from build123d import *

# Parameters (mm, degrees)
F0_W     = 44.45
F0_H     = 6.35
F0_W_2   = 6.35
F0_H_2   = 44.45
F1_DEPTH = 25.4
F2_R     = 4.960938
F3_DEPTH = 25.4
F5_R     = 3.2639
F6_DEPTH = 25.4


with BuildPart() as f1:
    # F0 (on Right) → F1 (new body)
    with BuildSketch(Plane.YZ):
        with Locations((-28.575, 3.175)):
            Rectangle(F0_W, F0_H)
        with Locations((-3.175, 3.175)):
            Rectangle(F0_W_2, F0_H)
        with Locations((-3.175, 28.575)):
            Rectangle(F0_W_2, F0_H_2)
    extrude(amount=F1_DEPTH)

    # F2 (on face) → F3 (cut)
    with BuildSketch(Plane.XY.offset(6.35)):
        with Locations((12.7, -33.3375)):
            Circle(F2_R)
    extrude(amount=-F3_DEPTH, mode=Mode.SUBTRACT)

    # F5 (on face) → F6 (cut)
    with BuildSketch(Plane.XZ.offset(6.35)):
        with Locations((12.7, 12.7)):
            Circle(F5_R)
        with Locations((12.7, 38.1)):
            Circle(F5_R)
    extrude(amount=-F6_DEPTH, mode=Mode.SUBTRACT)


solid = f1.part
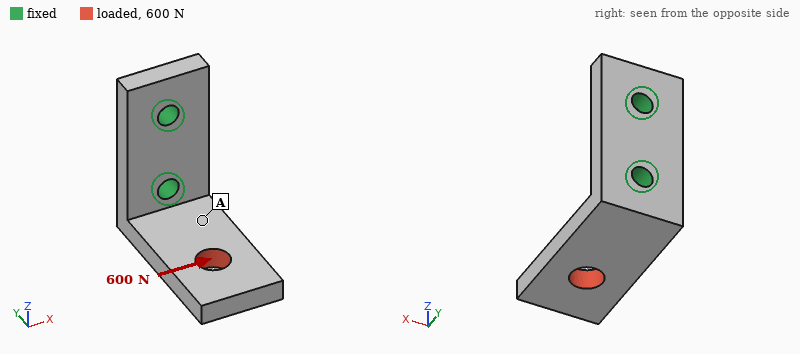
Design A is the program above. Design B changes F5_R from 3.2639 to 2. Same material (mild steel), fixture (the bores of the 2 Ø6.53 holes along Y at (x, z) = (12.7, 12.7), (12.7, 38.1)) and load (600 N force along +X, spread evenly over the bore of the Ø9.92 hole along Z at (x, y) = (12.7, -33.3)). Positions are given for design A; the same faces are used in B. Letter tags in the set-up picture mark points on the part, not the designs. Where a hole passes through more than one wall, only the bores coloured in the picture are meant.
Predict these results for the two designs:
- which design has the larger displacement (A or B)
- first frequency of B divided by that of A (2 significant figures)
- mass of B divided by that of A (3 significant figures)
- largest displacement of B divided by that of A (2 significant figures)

B
0.95
1.02
1.4
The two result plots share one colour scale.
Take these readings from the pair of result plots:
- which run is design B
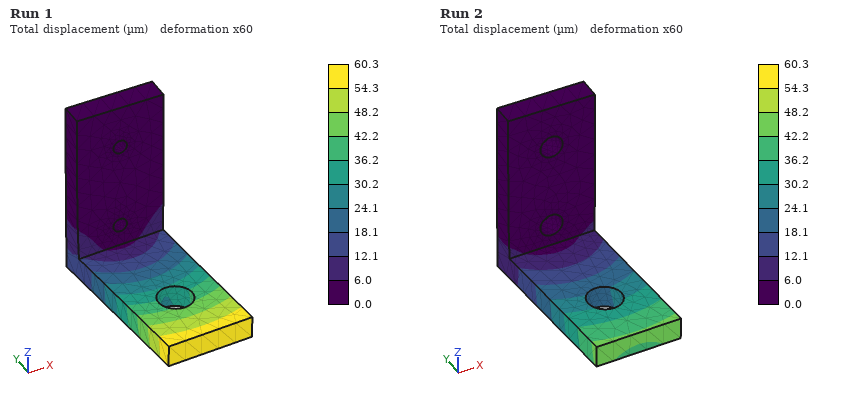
Run 1
